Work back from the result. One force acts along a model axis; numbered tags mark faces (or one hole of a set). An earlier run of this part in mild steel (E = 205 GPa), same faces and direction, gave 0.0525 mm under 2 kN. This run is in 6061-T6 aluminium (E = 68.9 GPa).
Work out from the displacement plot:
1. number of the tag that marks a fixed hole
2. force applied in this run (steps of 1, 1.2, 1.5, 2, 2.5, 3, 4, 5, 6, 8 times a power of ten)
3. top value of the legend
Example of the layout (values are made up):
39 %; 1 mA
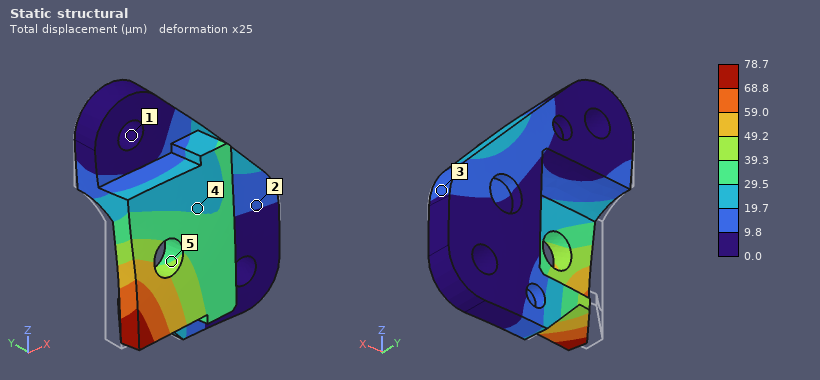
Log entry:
1; 1 kN; 78.7 µm
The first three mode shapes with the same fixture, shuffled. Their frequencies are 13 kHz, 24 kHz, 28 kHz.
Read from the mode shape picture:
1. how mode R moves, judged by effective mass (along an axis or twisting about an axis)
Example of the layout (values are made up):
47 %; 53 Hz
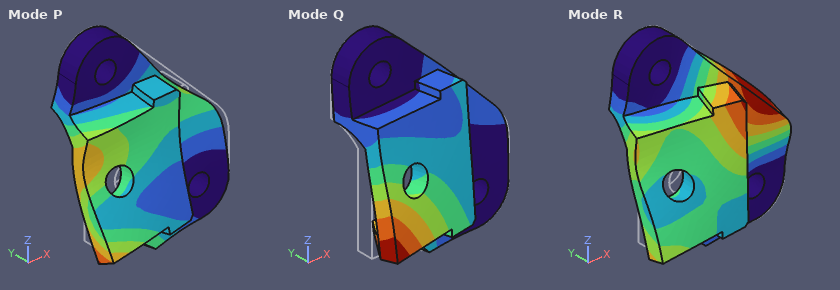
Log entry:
along Y
